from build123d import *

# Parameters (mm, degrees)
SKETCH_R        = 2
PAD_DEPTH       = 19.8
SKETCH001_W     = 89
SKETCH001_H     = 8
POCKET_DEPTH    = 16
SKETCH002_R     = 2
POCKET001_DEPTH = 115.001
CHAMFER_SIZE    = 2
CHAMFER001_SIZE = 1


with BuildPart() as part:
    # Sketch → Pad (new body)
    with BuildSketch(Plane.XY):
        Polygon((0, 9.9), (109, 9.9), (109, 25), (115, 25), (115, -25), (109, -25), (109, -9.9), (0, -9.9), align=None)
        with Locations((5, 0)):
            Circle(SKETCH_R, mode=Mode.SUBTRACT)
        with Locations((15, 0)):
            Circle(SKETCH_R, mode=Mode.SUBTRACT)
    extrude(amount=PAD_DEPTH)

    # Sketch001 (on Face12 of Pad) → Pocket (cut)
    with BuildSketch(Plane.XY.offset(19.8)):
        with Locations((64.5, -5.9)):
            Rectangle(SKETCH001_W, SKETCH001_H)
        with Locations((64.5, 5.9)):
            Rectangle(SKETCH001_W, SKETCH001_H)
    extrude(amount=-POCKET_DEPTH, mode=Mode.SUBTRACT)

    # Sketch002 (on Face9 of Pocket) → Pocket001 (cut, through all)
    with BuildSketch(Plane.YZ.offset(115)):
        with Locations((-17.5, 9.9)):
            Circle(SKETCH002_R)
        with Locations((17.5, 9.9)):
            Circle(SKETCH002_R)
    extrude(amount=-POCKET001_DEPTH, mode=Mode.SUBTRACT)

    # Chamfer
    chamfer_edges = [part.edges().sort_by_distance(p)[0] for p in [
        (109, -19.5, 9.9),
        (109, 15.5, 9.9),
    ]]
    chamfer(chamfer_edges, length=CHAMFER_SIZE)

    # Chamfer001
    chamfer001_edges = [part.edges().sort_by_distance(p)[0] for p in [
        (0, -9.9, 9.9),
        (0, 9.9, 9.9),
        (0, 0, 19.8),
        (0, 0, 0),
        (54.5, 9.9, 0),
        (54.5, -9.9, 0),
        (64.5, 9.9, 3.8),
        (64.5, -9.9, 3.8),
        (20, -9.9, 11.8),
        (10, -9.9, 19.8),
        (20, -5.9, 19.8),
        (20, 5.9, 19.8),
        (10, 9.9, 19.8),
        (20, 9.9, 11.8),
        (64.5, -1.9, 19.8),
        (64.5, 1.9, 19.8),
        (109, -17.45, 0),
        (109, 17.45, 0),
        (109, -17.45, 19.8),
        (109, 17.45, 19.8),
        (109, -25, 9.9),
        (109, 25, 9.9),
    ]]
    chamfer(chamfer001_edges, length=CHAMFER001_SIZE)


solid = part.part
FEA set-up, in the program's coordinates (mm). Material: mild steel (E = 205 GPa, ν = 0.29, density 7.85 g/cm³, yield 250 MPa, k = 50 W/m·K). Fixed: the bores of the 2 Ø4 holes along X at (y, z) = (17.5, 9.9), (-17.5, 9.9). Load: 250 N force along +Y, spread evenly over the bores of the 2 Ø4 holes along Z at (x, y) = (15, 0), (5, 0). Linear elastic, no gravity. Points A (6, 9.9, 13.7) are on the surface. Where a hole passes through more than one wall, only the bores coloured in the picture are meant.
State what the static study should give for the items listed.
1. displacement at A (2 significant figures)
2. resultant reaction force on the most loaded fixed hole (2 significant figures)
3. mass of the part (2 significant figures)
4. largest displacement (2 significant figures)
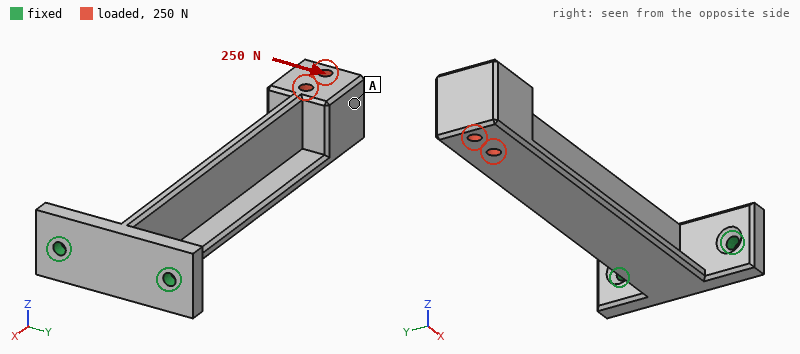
0.30 mm
900 N
190 g
0.33 mm
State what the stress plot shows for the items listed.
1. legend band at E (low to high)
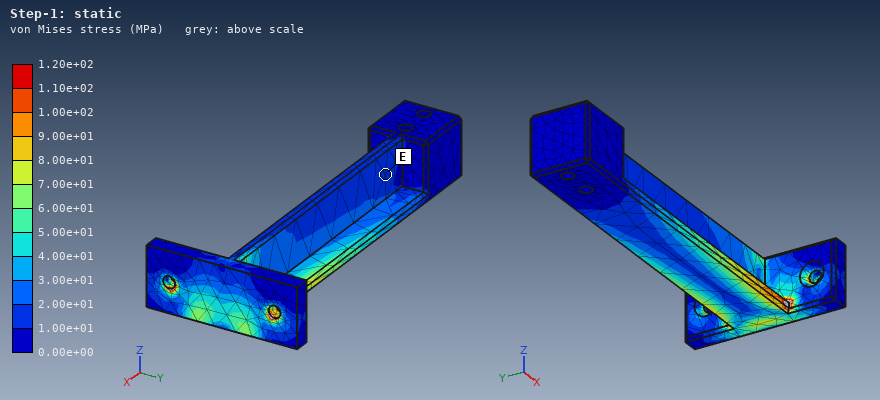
1.00e+01 to 2.00e+01 MPa
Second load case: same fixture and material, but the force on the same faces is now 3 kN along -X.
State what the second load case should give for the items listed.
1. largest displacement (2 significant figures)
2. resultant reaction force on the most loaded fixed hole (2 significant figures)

0.12 mm
1.7 kN
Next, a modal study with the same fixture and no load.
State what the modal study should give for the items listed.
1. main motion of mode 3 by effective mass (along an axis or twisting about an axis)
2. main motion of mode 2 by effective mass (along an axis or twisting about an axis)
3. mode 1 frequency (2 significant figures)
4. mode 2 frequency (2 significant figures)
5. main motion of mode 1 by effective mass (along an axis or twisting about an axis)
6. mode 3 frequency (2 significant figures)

twisting about X
along Y
500 Hz
560 Hz
along Z
1800 Hz
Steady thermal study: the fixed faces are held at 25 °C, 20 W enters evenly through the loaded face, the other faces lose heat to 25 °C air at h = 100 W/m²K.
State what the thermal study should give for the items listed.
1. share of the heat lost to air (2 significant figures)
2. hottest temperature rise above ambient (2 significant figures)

97 %
53 K
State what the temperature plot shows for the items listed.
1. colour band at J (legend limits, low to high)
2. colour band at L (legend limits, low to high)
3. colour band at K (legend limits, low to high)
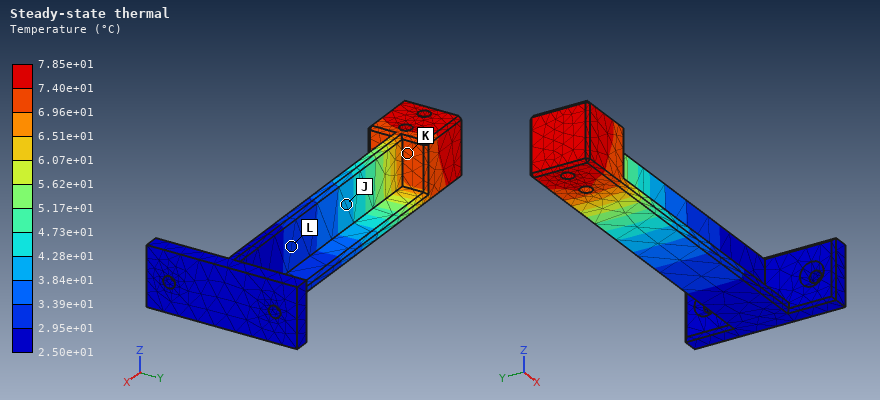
3.84e+01 to 4.28e+01 °C
2.95e+01 to 3.39e+01 °C
6.96e+01 to 7.40e+01 °C
